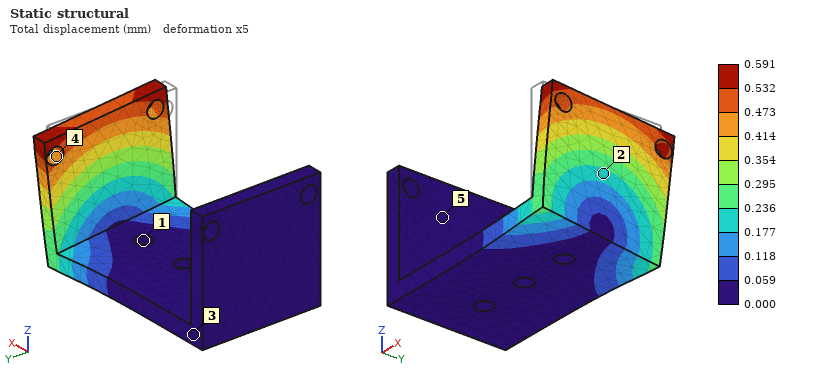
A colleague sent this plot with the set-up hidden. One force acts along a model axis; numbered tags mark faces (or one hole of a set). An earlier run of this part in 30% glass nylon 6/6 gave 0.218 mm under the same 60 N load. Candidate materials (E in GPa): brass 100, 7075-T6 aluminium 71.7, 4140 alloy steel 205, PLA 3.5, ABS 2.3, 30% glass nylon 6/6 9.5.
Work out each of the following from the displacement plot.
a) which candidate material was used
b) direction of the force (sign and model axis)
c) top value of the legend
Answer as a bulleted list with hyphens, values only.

- PLA
- +Y
- 0.591 mm
